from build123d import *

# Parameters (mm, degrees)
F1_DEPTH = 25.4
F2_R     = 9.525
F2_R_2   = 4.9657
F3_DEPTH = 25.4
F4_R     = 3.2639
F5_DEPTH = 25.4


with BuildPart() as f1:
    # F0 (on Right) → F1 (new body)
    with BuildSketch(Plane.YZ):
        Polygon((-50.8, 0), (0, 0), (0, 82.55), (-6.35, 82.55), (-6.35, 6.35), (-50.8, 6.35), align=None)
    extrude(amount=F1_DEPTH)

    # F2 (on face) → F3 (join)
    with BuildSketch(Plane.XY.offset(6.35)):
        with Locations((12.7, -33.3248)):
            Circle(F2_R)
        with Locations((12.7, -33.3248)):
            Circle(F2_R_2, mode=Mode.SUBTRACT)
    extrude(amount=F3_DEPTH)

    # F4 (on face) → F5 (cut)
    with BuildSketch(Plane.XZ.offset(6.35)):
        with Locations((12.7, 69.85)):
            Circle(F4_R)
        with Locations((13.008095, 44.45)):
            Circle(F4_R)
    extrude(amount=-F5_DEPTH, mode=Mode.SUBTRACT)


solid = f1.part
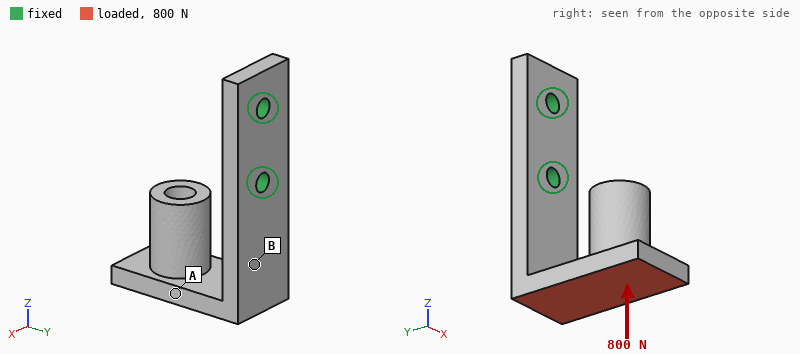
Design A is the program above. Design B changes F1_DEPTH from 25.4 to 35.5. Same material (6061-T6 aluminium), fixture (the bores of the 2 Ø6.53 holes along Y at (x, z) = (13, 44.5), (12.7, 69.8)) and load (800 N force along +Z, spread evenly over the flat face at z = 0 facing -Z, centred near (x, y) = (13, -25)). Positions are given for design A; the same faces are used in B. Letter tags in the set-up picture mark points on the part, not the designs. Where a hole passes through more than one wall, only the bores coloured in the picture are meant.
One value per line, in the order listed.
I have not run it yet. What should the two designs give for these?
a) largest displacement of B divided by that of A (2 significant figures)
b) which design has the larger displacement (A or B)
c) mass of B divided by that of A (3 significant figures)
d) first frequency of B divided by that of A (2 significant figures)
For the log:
0.73
A
1.32
1.0
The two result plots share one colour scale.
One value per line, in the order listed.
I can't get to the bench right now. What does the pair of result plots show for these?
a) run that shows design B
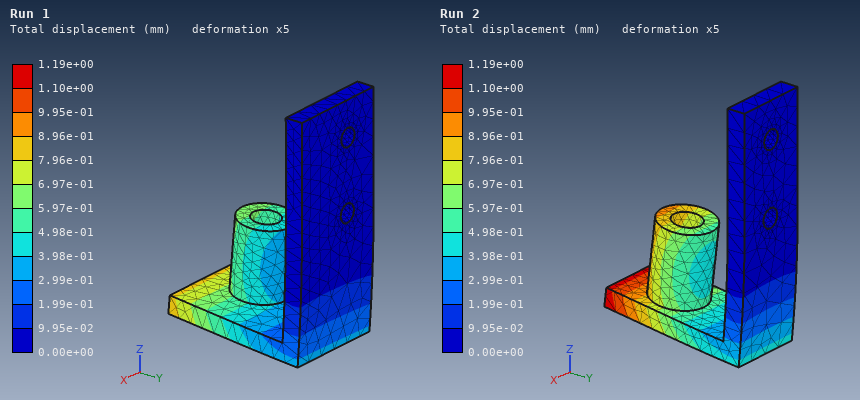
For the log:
Run 1
